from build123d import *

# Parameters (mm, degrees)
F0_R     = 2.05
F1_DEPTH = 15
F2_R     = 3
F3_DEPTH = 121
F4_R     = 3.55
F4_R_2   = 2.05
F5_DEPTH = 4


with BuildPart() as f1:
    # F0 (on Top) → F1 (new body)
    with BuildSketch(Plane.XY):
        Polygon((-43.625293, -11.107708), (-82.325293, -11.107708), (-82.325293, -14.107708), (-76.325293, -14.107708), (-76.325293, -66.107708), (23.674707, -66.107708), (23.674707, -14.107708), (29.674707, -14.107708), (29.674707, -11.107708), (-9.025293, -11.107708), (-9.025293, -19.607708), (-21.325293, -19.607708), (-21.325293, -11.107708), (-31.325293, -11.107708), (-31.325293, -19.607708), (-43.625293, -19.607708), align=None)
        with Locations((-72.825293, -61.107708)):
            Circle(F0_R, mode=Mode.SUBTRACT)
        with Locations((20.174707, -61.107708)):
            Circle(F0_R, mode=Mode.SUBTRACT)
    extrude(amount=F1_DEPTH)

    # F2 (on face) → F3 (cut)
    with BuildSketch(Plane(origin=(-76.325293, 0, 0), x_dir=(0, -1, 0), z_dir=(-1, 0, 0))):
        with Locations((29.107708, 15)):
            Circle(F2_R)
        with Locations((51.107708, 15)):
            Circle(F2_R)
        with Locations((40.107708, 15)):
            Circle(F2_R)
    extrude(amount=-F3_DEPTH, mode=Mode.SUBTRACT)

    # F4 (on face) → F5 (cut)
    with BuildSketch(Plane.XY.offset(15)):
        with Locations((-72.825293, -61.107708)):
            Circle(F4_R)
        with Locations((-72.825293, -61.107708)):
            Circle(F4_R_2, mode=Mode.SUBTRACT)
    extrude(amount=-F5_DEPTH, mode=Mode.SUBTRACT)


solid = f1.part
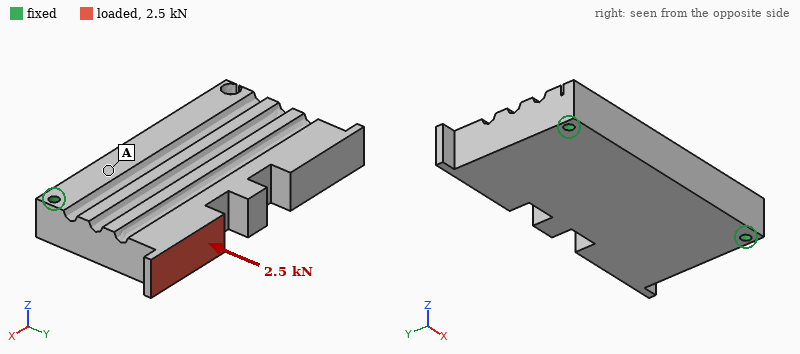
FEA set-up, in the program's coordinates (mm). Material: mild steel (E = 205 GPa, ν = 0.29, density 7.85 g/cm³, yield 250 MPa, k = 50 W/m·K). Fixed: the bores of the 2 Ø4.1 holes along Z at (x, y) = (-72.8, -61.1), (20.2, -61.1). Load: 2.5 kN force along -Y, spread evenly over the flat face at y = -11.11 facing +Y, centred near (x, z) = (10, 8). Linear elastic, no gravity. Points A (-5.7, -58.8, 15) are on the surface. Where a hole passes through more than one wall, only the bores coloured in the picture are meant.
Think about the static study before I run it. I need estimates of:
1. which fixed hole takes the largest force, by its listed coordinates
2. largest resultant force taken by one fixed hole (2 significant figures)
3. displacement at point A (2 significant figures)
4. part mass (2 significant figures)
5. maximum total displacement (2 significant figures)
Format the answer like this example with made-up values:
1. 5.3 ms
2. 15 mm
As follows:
1. (20.2, -61.1)
2. 2.3 kN
3. 1.4 µm
4. 590 g
5. 8.1 µm
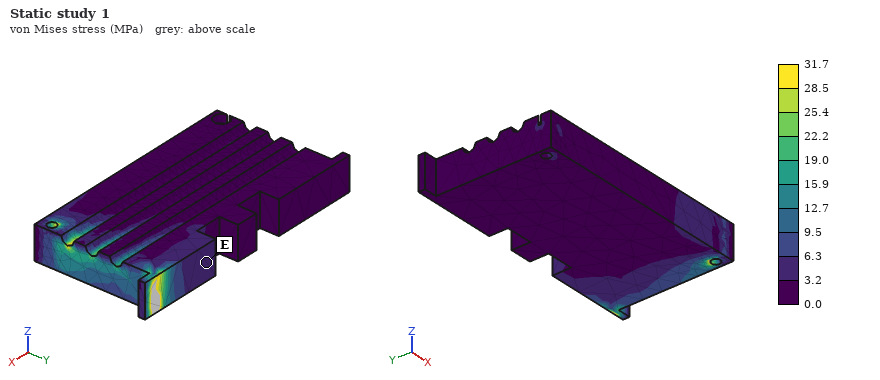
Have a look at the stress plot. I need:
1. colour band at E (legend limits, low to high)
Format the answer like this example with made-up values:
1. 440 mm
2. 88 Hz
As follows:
1. 3.2 to 6.3 MPa
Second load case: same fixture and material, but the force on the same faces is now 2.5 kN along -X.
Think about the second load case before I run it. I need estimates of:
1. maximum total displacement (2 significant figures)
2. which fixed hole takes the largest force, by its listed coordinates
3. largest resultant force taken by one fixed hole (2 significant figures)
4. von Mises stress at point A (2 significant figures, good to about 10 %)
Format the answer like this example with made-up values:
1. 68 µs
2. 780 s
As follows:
1. 9.4 µm
2. (-72.8, -61.1)
3. 2.1 kN
4. 2.9 MPa
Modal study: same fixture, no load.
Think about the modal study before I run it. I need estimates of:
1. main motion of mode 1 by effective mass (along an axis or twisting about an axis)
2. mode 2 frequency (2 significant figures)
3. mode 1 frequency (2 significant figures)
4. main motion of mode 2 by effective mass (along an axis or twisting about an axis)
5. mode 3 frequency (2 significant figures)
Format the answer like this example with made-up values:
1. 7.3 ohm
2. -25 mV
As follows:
1. along Z
2. 4800 Hz
3. 2200 Hz
4. twisting about Y
5. 6500 Hz
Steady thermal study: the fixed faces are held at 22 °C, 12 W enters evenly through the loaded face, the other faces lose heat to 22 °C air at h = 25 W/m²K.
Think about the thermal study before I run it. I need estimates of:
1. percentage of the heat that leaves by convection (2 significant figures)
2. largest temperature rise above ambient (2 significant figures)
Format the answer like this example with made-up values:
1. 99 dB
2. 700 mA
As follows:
1. 24 %
2. 27 K
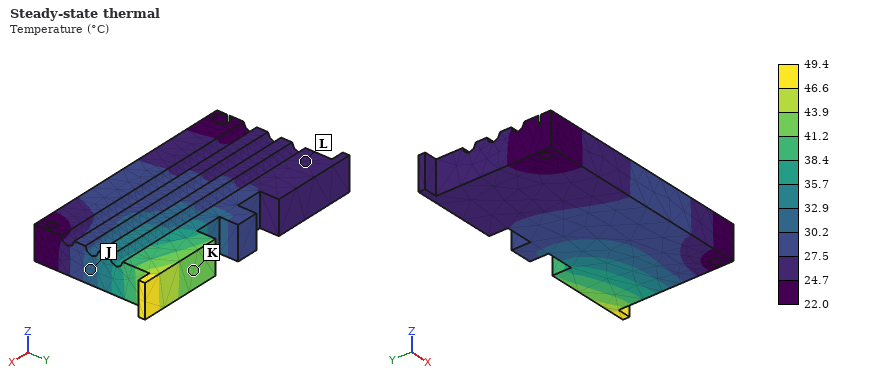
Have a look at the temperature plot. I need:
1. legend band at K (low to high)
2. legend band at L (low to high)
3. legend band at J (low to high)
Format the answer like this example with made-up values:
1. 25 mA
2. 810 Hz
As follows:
1. 41.2 to 43.9 °C
2. 24.7 to 27.5 °C
3. 30.2 to 32.9 °C
